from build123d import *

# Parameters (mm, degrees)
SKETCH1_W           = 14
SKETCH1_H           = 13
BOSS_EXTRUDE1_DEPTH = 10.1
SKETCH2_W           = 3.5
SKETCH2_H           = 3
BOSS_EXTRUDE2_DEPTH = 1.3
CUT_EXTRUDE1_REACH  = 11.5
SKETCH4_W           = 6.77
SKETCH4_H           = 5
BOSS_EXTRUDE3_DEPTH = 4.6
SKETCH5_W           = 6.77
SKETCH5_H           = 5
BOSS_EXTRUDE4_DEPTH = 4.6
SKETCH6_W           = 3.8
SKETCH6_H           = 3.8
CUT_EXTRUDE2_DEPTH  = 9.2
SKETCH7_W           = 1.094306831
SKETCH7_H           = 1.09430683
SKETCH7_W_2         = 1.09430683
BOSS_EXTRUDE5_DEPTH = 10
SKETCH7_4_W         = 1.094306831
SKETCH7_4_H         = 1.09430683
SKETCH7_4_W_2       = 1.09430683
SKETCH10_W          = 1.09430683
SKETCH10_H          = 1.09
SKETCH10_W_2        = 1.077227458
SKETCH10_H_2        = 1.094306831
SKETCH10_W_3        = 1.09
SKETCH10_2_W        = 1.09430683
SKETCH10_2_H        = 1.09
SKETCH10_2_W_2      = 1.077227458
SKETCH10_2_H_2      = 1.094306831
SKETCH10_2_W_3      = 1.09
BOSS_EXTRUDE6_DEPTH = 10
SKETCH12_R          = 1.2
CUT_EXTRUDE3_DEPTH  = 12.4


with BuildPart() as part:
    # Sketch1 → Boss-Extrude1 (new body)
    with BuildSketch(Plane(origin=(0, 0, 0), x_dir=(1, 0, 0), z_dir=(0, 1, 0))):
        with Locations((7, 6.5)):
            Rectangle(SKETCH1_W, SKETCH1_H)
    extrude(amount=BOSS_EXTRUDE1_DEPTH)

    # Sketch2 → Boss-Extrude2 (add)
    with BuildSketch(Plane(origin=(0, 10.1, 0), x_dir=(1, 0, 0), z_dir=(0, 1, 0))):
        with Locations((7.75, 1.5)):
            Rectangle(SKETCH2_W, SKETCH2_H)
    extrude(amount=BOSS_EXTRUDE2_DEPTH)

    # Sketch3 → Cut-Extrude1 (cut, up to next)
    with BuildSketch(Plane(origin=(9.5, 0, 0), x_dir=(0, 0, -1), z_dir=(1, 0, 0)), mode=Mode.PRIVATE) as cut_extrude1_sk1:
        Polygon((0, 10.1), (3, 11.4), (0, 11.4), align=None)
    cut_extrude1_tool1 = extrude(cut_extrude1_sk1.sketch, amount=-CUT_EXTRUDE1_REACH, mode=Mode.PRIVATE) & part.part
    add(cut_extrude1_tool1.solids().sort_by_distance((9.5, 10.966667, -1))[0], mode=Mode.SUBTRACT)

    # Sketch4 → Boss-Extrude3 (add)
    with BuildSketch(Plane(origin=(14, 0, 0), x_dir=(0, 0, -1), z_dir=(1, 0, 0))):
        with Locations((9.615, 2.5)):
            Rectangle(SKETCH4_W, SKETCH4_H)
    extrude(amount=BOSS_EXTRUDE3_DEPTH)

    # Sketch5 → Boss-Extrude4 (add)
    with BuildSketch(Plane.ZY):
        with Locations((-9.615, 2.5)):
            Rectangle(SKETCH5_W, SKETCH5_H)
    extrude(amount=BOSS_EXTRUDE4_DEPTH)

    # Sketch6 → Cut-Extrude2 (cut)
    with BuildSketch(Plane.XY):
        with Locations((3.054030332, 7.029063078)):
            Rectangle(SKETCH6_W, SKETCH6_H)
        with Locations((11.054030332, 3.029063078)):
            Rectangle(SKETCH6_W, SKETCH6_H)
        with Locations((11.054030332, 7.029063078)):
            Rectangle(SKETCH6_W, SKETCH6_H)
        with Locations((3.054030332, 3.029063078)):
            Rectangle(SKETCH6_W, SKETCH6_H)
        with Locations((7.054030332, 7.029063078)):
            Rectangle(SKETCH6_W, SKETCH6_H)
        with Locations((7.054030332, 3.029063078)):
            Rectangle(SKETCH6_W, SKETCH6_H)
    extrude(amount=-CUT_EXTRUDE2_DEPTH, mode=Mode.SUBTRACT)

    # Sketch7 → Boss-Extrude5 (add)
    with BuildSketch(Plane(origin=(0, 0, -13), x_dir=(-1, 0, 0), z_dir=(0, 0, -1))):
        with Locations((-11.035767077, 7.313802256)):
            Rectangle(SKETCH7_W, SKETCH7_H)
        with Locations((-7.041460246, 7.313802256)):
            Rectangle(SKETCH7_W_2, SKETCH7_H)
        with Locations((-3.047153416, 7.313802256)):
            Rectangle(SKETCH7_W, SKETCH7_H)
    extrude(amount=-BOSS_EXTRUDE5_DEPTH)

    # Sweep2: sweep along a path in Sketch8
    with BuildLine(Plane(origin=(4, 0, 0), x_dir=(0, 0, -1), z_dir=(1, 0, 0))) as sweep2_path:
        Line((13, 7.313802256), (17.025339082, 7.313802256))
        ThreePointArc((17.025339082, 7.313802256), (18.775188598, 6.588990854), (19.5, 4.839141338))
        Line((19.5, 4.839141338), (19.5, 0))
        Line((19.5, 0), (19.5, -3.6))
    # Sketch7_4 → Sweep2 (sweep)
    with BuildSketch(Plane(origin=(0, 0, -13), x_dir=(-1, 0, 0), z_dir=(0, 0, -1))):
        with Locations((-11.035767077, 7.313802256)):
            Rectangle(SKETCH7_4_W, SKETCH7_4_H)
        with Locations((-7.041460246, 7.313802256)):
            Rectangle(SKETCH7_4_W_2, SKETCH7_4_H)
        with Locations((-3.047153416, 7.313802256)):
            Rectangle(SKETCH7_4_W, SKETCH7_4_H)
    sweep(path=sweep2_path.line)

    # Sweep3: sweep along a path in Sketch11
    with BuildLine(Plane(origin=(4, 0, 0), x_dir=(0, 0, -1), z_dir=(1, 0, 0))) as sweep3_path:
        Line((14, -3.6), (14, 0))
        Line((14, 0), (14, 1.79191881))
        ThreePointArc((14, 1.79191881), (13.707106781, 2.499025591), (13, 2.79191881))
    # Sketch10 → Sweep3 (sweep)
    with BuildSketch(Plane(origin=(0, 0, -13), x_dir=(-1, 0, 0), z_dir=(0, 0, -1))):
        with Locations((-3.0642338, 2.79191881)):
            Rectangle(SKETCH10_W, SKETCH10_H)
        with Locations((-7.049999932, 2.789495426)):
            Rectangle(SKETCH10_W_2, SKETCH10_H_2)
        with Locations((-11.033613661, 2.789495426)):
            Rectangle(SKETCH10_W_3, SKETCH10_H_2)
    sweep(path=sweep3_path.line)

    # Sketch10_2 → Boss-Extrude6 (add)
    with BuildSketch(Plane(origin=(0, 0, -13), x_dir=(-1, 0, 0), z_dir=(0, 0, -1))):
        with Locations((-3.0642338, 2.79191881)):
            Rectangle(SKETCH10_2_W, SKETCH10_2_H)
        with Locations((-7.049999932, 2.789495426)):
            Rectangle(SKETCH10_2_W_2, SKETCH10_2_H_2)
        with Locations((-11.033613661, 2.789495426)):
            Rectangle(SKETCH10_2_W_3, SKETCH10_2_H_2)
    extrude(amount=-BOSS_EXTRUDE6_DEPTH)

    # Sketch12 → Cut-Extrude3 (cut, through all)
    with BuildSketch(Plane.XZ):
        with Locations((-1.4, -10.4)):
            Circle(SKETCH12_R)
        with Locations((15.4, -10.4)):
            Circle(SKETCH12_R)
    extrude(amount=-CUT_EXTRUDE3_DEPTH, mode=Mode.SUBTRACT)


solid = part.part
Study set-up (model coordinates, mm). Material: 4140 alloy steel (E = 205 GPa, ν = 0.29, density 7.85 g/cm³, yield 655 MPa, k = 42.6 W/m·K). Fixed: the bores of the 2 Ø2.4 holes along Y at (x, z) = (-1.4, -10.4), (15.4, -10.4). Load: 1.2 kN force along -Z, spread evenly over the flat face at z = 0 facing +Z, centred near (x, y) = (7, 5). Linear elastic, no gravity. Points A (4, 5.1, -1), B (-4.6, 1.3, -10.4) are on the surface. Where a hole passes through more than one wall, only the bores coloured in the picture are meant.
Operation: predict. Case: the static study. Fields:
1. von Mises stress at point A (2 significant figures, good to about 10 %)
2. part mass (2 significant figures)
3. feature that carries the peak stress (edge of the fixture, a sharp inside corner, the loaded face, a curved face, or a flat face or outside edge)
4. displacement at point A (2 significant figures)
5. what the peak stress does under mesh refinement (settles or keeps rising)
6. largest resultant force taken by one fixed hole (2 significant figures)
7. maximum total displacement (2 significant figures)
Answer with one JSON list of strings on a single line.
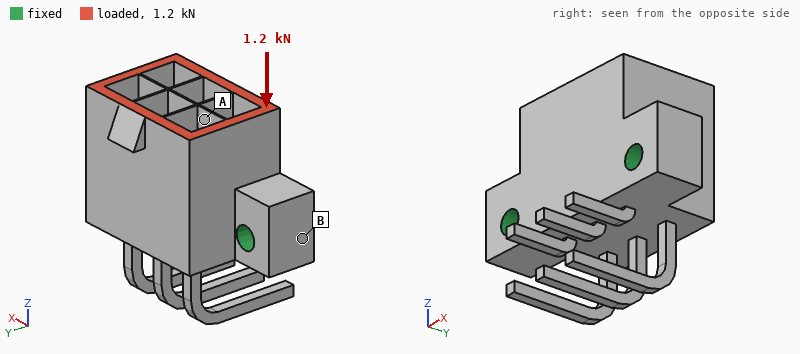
["23 MPa", "11 g", "edge of the fixture", "4.5 µm", "keeps rising", "610 N", "6.6 µm"]
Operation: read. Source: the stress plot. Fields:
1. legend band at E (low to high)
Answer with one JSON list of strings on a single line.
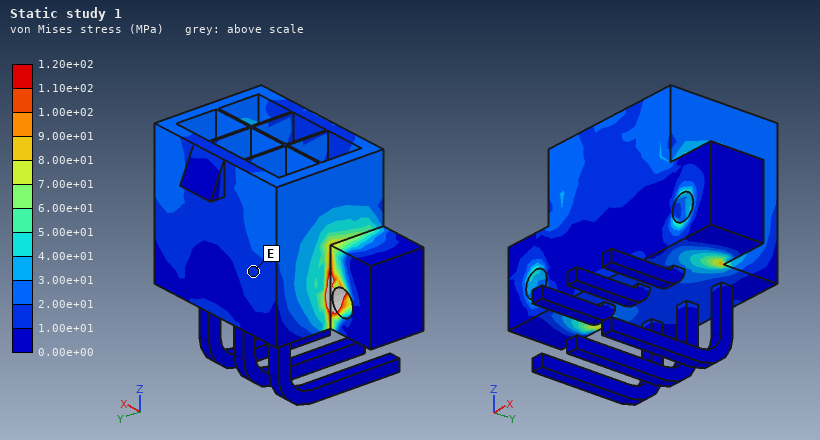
["1.00e+01 to 2.00e+01 MPa"]
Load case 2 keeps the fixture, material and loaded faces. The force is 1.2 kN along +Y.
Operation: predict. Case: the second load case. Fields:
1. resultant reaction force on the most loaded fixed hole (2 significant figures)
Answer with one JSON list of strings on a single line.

["630 N"]
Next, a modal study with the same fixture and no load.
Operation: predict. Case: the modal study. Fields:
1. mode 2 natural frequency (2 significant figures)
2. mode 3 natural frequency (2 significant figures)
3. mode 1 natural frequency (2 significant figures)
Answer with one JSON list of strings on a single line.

["3500 Hz", "3500 Hz", "3500 Hz"]
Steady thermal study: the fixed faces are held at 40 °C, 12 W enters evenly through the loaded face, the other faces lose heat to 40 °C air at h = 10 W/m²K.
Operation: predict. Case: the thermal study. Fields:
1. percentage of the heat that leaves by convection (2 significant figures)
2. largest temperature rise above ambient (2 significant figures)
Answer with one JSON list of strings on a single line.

["4.5 %", "59 K"]
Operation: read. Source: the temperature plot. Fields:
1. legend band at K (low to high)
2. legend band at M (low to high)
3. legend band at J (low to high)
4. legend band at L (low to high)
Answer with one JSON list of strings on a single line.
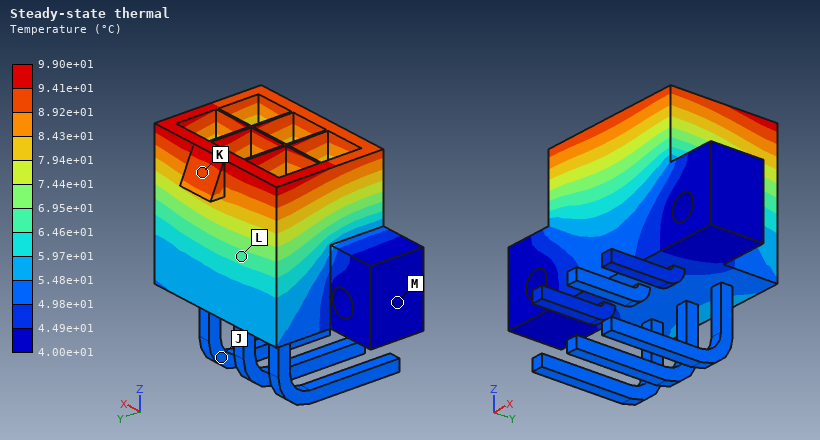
["8.92e+01 to 9.41e+01 °C", "4.00e+01 to 4.49e+01 °C", "4.98e+01 to 5.48e+01 °C", "6.46e+01 to 6.95e+01 °C"]
